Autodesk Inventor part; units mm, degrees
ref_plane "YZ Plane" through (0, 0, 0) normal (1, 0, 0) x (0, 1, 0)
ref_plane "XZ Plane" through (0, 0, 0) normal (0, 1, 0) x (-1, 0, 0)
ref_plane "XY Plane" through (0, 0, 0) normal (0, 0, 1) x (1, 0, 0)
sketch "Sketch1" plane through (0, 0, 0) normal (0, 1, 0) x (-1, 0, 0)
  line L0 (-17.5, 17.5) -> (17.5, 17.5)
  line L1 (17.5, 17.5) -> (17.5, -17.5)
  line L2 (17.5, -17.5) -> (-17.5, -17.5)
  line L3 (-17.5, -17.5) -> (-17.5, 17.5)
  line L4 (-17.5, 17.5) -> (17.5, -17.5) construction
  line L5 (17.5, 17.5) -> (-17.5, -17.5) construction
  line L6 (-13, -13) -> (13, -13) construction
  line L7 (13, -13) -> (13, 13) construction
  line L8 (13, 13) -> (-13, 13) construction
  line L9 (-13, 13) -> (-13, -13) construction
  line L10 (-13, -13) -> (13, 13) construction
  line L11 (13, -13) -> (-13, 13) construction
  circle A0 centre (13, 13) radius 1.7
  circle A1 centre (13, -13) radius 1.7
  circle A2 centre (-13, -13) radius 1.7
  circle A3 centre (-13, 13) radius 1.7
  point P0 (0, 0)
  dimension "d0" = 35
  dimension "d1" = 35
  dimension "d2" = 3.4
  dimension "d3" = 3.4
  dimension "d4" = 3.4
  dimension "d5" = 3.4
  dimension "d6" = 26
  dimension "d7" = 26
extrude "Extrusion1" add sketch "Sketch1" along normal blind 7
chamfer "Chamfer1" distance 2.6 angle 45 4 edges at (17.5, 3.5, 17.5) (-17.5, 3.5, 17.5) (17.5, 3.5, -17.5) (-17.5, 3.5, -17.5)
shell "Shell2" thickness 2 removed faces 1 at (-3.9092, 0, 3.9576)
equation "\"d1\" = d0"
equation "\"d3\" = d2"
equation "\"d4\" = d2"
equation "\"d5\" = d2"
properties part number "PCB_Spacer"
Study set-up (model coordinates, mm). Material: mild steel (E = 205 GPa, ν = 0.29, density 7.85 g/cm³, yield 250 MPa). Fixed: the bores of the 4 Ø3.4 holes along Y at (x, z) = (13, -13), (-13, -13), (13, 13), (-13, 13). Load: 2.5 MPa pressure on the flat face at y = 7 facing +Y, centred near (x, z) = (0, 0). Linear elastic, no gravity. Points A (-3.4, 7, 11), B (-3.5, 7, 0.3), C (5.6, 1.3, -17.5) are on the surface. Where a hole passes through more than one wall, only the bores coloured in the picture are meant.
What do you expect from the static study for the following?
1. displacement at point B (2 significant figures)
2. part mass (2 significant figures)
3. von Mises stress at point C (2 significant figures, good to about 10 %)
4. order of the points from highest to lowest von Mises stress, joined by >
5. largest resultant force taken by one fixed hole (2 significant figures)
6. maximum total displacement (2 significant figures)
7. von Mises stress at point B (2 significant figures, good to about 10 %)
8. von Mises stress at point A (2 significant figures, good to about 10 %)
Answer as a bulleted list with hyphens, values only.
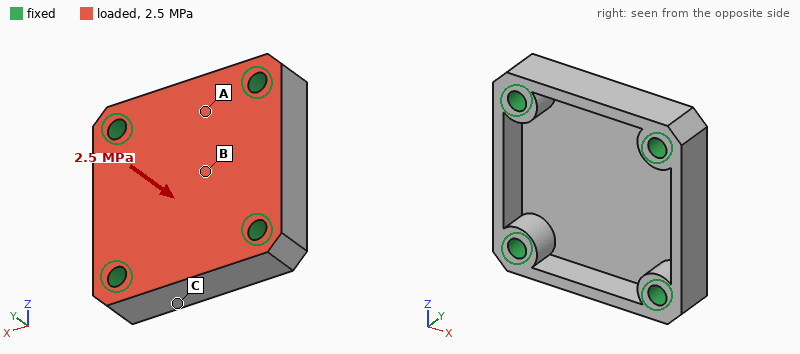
- 25 µm
- 32 g
- 17 MPa
- B > A > C
- 760 N
- 26 µm
- 87 MPa
- 55 MPa
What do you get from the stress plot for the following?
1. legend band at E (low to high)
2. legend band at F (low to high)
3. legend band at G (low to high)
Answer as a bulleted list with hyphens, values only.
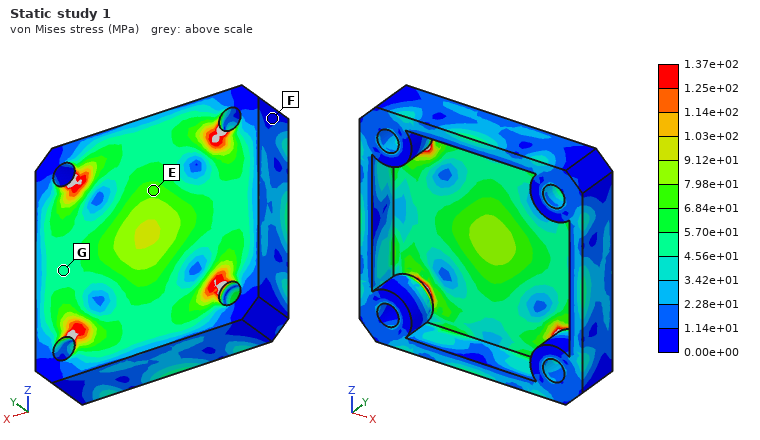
- 6.84e+01 to 7.98e+01 MPa
- 0.00e+00 to 1.14e+01 MPa
- 4.56e+01 to 5.70e+01 MPa
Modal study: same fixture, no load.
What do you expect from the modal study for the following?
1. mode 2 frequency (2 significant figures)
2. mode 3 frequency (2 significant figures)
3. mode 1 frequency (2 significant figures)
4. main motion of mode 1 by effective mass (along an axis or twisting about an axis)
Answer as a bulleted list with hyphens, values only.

- 29 kHz
- 29 kHz
- 15 kHz
- along Y
